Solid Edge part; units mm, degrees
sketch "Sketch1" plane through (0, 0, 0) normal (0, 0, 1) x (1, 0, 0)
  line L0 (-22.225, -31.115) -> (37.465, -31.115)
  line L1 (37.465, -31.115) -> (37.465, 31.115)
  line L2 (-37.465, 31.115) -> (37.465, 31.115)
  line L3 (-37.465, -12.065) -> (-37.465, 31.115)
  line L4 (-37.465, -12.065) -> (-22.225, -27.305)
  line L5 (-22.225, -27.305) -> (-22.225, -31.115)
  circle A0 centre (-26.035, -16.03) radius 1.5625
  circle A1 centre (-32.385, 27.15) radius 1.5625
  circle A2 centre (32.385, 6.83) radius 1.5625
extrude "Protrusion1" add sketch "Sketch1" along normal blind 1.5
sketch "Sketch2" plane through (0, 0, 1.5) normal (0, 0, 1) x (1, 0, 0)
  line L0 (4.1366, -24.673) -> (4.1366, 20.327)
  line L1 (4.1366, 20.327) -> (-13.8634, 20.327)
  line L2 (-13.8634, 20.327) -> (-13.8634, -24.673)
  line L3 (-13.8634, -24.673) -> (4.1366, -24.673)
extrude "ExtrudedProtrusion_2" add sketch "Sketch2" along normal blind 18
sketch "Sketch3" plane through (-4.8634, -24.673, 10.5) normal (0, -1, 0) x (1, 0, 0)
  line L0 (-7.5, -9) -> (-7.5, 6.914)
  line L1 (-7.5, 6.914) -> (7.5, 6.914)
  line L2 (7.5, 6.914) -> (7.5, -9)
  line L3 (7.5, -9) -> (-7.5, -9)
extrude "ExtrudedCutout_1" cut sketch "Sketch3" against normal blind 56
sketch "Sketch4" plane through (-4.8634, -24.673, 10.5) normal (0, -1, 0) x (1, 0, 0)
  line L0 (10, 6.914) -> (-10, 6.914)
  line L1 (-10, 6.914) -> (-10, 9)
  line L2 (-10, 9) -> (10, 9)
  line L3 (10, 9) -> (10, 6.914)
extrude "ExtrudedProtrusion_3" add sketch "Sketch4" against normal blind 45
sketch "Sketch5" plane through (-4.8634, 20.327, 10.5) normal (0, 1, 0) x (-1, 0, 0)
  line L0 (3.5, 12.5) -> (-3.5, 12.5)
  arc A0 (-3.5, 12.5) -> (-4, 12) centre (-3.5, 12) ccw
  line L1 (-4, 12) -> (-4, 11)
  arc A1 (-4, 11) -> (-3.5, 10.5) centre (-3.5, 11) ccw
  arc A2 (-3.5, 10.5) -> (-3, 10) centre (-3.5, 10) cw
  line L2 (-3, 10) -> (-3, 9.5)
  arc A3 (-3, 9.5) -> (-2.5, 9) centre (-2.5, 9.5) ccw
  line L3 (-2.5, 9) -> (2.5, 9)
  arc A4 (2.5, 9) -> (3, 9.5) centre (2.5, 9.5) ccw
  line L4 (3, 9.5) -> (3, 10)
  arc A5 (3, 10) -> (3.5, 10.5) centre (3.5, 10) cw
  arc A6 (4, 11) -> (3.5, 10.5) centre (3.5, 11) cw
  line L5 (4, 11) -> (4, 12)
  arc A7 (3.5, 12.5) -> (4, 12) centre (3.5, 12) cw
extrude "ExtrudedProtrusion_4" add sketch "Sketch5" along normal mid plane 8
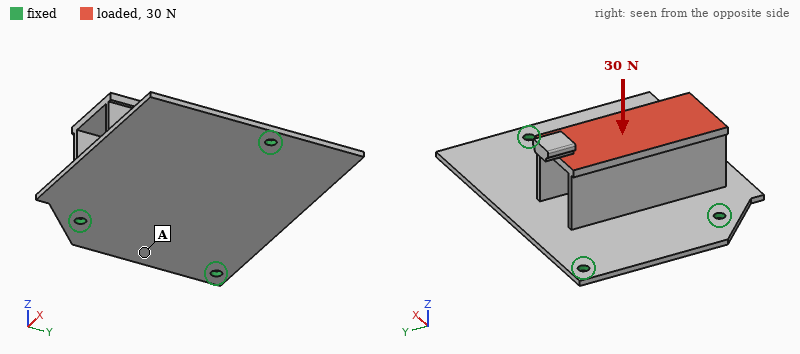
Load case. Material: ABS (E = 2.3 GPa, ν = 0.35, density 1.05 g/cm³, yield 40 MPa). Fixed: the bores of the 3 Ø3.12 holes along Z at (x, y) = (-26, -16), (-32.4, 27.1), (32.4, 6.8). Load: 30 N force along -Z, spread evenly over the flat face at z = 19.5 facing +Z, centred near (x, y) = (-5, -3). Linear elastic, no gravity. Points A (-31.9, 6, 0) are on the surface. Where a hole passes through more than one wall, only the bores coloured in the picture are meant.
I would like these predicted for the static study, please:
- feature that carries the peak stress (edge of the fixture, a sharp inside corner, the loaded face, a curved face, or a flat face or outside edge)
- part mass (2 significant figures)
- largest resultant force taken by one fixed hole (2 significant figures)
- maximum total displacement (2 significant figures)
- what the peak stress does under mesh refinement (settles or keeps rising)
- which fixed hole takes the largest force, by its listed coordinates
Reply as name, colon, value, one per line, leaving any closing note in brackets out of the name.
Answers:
feature that carries the peak stress: edge of the fixture
part mass: 11 g
largest resultant force taken by one fixed hole: 16 N
maximum total displacement: 0.88 mm
what the peak stress does under mesh refinement: keeps rising
which fixed hole takes the largest force, by its listed coordinates: (-26, -16)
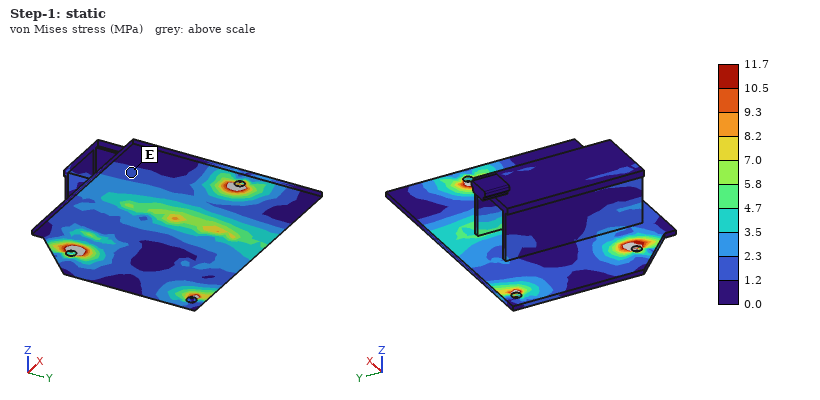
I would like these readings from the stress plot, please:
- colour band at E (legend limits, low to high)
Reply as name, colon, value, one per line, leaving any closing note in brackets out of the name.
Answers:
colour band at E: 1.2 to 2.3 MPa
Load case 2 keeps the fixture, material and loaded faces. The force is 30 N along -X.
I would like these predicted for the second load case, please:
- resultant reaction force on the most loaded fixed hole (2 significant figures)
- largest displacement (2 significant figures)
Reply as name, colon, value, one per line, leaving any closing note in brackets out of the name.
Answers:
resultant reaction force on the most loaded fixed hole: 15 N
largest displacement: 1.0 mm
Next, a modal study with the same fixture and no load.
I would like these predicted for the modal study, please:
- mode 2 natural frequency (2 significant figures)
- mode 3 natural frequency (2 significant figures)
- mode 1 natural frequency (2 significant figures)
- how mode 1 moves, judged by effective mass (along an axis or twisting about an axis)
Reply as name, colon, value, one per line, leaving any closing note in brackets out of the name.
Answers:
mode 2 natural frequency: 380 Hz
mode 3 natural frequency: 610 Hz
mode 1 natural frequency: 330 Hz
how mode 1 moves, judged by effective mass: along Z
